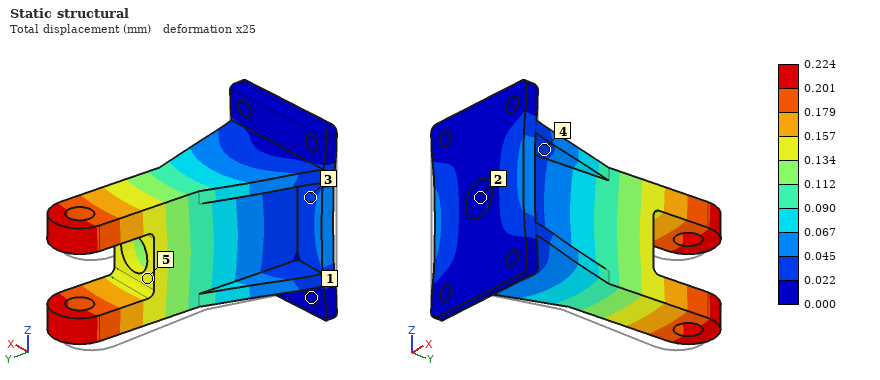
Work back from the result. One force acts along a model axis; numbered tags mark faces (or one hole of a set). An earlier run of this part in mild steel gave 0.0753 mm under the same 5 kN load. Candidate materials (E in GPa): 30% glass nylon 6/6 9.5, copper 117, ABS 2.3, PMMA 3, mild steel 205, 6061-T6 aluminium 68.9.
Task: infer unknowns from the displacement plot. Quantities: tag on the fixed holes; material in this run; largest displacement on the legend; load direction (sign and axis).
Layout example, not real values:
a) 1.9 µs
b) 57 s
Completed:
a) 1
b) 6061-T6 aluminium
c) 0.224 mm
d) +X
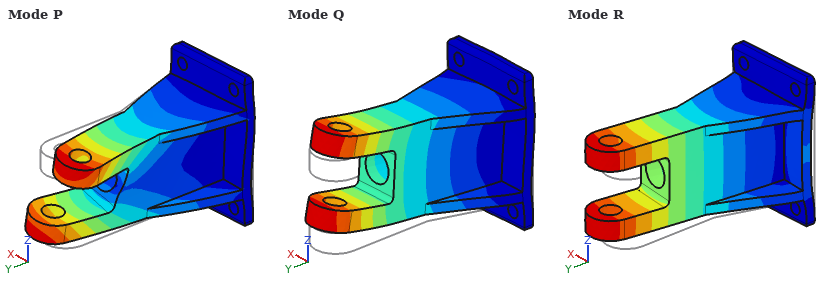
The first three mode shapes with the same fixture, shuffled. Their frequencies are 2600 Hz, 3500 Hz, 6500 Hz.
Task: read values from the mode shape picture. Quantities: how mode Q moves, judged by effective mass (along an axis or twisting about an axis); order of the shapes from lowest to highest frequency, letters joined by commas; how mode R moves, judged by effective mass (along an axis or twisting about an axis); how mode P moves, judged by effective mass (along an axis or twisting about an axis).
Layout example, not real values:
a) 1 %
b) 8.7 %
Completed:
a) along Z
b) R, Q, P
c) along X
d) twisting about Y
